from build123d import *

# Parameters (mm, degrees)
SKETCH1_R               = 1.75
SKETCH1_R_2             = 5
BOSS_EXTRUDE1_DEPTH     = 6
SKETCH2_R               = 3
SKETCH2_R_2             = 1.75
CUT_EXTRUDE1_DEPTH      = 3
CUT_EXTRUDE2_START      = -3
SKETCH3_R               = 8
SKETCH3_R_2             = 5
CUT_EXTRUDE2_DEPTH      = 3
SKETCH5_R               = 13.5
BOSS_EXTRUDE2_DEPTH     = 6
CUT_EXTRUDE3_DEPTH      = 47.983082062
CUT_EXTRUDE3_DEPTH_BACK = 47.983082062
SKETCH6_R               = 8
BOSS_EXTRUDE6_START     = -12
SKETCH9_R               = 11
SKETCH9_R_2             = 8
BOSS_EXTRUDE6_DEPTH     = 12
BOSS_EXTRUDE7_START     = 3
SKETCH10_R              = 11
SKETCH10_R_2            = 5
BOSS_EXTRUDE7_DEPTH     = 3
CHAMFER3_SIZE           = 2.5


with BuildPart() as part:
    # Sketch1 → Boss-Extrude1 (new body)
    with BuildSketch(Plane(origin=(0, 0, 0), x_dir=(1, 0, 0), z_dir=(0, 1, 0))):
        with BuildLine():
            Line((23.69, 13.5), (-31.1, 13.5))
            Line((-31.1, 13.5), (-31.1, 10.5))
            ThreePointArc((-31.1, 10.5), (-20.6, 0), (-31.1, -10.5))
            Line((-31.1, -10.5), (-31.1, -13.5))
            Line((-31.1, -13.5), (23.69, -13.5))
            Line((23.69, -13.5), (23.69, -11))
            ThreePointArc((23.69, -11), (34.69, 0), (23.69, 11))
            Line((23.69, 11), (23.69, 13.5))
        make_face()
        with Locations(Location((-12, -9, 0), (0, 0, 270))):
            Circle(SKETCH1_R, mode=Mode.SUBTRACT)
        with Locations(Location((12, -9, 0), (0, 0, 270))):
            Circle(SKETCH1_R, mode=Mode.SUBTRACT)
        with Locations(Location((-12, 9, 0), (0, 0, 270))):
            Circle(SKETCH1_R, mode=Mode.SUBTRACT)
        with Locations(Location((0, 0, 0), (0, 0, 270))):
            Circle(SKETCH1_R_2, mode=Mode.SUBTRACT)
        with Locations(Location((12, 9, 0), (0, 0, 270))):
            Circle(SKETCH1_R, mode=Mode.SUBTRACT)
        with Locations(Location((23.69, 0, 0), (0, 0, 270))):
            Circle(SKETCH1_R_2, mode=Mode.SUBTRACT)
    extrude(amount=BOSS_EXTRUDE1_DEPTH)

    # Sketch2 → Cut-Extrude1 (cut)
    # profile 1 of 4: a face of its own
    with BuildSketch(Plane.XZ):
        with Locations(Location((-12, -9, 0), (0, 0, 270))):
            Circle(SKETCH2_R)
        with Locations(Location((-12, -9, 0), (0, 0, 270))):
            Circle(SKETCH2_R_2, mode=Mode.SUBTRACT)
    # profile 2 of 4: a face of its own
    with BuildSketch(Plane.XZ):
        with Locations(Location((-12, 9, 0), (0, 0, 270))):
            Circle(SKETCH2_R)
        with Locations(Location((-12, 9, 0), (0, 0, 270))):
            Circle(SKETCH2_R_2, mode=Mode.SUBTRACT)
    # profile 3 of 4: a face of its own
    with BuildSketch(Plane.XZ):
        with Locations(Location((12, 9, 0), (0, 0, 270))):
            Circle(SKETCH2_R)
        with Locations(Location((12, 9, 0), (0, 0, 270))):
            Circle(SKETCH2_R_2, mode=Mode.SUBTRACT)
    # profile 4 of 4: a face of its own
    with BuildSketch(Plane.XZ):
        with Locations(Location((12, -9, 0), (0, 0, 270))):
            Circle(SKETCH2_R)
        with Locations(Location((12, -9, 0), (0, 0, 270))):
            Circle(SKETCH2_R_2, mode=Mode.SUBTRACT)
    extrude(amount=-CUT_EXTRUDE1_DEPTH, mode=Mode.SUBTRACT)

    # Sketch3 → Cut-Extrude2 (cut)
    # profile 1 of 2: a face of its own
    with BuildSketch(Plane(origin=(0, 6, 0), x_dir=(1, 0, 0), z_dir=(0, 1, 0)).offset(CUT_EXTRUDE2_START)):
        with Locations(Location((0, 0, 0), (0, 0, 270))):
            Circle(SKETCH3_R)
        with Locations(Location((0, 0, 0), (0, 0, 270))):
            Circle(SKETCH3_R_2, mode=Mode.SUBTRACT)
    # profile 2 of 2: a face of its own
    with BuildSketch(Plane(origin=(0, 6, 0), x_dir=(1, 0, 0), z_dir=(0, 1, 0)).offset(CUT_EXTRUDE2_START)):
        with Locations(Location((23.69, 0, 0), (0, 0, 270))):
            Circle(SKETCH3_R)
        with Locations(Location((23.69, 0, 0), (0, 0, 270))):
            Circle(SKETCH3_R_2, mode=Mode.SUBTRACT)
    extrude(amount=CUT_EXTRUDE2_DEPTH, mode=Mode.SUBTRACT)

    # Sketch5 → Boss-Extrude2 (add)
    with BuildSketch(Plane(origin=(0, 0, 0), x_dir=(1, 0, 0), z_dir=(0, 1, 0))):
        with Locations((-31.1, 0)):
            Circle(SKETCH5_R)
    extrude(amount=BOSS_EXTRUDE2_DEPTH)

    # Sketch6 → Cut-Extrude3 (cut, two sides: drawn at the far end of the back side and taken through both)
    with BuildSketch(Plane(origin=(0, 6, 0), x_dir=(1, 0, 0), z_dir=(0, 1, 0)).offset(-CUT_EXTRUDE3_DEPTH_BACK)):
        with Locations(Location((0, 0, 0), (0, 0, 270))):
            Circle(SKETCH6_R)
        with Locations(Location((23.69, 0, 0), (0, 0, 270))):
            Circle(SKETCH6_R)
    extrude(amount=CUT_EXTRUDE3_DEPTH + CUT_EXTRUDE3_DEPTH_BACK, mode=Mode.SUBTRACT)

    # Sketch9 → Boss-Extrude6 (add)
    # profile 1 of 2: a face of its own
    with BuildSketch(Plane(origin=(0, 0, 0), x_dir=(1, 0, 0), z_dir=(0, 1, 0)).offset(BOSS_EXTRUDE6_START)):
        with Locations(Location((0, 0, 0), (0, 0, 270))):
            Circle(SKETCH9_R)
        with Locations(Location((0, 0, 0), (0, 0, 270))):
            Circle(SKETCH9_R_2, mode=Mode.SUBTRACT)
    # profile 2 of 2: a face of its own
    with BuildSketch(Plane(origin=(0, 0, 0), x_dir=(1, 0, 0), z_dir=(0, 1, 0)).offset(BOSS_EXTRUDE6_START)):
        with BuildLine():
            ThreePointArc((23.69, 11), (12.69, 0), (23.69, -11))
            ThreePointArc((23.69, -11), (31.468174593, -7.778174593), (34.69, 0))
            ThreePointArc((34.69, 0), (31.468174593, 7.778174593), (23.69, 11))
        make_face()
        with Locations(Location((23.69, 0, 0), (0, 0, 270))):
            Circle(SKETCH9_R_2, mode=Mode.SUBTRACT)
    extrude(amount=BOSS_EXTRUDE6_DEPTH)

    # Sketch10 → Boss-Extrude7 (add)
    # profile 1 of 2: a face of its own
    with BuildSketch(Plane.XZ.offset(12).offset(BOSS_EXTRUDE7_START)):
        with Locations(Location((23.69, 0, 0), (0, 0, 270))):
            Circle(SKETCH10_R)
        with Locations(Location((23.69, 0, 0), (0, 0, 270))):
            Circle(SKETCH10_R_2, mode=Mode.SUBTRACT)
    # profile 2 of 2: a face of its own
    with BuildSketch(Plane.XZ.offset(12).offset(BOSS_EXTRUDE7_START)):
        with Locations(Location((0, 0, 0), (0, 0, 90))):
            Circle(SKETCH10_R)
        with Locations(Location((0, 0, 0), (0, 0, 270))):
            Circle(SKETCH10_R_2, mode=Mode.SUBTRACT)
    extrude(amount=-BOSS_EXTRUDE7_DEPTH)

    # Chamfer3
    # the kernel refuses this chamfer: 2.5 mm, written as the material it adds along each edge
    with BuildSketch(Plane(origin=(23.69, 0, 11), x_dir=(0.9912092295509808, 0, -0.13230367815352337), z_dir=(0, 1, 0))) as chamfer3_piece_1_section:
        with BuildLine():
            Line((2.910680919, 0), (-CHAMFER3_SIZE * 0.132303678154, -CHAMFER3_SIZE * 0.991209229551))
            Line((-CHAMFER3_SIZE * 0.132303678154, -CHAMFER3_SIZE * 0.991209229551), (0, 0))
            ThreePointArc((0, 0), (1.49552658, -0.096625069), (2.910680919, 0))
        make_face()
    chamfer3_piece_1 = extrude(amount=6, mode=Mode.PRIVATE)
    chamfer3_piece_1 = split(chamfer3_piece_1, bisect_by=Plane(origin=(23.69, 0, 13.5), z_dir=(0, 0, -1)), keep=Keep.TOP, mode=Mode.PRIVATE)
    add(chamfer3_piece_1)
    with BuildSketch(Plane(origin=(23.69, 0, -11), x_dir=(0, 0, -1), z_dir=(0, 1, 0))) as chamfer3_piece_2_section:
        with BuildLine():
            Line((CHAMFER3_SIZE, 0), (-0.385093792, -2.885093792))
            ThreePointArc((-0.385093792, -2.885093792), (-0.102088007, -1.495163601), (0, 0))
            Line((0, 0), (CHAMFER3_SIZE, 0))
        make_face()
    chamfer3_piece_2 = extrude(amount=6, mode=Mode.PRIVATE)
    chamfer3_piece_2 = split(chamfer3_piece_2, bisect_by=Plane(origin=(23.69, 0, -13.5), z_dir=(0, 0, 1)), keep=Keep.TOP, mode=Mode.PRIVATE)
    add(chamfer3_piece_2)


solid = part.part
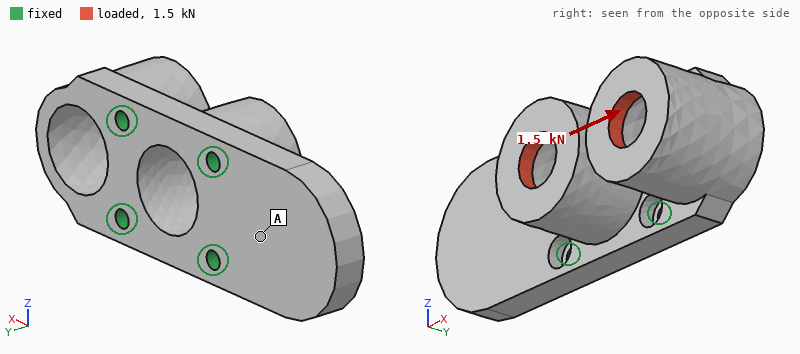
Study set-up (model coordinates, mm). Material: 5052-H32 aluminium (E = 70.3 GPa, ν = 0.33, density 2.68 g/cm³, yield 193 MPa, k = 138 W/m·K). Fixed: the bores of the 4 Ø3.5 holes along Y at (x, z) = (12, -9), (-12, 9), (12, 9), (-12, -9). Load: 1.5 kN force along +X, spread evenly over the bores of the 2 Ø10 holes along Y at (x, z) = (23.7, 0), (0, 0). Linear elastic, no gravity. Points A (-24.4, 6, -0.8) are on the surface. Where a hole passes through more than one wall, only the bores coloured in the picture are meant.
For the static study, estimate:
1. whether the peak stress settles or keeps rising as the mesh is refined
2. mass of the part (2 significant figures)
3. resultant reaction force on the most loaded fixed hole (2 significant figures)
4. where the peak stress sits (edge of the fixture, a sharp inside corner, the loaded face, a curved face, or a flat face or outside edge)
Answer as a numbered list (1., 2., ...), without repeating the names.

1. keeps rising
2. 40 g
3. 660 N
4. edge of the fixture
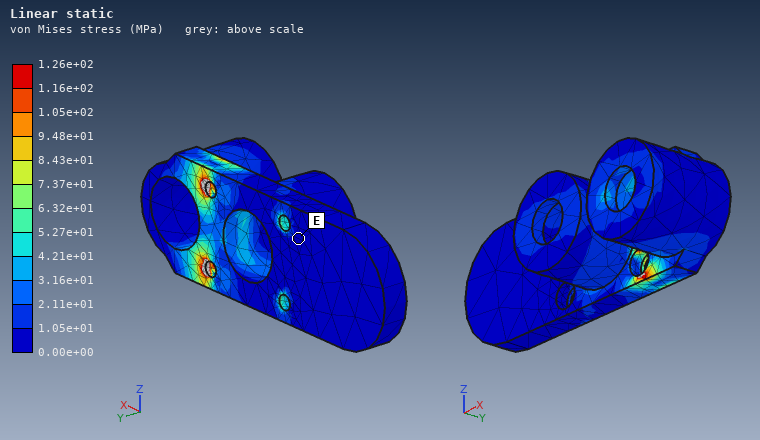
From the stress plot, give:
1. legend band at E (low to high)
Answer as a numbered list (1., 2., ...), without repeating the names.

1. 0.00e+00 to 1.05e+01 MPa
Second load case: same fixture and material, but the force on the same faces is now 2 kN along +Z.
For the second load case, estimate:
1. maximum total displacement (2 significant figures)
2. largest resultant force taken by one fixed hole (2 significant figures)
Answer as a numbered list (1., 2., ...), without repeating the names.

1. 40 µm
2. 1.7 kN
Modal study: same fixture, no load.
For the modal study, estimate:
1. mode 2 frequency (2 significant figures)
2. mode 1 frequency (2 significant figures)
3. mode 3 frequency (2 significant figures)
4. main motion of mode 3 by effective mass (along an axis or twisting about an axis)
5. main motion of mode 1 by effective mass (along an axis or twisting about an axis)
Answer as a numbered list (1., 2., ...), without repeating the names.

1. 4800 Hz
2. 4300 Hz
3. 11 kHz
4. along Z
5. along Y
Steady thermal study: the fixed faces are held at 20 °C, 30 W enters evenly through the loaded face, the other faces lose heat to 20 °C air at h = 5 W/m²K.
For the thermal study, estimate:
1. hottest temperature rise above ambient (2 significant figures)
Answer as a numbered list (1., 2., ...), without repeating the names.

1. 23 K
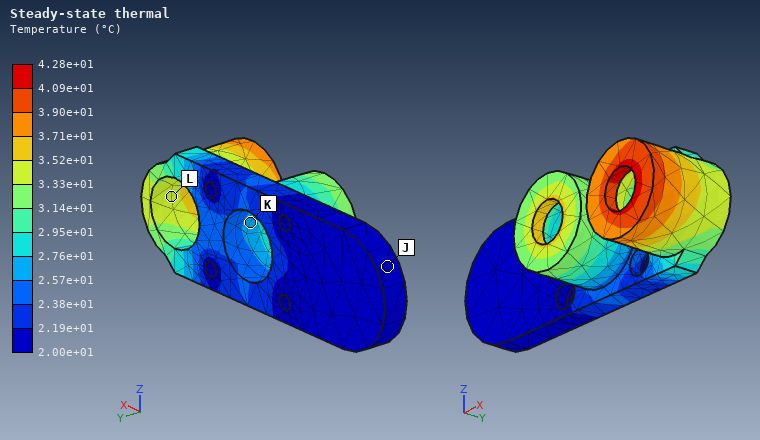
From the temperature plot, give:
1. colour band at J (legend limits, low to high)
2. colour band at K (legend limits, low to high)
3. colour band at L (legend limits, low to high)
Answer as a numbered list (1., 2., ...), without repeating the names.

1. 2.00e+01 to 2.19e+01 °C
2. 2.57e+01 to 2.76e+01 °C
3. 3.33e+01 to 3.52e+01 °C
